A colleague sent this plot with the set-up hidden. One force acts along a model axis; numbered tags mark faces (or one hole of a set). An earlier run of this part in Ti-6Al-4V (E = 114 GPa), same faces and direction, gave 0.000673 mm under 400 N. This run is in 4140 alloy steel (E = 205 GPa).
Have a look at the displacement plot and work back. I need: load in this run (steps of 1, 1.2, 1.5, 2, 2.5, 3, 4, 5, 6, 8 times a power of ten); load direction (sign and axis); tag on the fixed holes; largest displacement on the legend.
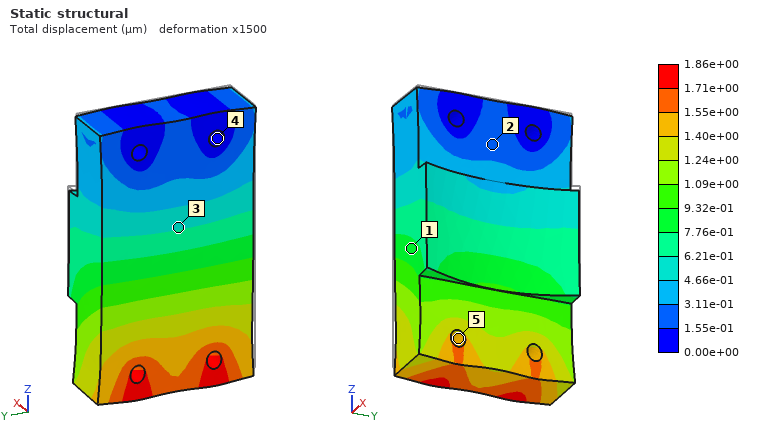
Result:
2 kN
-Z
4
1.86e+00 µm
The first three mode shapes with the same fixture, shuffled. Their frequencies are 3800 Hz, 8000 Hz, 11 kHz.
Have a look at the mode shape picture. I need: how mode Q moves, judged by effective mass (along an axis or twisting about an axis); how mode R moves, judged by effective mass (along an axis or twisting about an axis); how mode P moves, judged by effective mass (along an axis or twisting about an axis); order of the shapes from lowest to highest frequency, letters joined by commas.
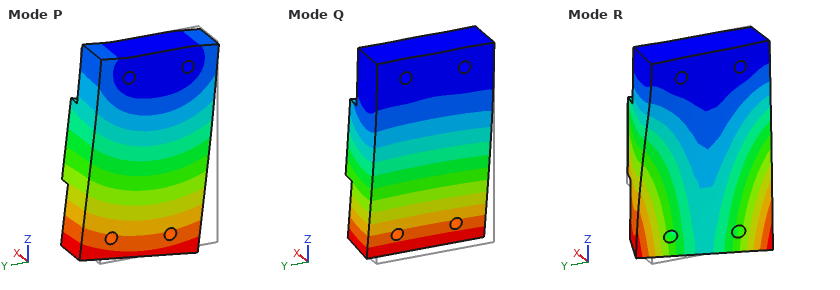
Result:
along X
twisting about Z
along Y
Q, P, R
